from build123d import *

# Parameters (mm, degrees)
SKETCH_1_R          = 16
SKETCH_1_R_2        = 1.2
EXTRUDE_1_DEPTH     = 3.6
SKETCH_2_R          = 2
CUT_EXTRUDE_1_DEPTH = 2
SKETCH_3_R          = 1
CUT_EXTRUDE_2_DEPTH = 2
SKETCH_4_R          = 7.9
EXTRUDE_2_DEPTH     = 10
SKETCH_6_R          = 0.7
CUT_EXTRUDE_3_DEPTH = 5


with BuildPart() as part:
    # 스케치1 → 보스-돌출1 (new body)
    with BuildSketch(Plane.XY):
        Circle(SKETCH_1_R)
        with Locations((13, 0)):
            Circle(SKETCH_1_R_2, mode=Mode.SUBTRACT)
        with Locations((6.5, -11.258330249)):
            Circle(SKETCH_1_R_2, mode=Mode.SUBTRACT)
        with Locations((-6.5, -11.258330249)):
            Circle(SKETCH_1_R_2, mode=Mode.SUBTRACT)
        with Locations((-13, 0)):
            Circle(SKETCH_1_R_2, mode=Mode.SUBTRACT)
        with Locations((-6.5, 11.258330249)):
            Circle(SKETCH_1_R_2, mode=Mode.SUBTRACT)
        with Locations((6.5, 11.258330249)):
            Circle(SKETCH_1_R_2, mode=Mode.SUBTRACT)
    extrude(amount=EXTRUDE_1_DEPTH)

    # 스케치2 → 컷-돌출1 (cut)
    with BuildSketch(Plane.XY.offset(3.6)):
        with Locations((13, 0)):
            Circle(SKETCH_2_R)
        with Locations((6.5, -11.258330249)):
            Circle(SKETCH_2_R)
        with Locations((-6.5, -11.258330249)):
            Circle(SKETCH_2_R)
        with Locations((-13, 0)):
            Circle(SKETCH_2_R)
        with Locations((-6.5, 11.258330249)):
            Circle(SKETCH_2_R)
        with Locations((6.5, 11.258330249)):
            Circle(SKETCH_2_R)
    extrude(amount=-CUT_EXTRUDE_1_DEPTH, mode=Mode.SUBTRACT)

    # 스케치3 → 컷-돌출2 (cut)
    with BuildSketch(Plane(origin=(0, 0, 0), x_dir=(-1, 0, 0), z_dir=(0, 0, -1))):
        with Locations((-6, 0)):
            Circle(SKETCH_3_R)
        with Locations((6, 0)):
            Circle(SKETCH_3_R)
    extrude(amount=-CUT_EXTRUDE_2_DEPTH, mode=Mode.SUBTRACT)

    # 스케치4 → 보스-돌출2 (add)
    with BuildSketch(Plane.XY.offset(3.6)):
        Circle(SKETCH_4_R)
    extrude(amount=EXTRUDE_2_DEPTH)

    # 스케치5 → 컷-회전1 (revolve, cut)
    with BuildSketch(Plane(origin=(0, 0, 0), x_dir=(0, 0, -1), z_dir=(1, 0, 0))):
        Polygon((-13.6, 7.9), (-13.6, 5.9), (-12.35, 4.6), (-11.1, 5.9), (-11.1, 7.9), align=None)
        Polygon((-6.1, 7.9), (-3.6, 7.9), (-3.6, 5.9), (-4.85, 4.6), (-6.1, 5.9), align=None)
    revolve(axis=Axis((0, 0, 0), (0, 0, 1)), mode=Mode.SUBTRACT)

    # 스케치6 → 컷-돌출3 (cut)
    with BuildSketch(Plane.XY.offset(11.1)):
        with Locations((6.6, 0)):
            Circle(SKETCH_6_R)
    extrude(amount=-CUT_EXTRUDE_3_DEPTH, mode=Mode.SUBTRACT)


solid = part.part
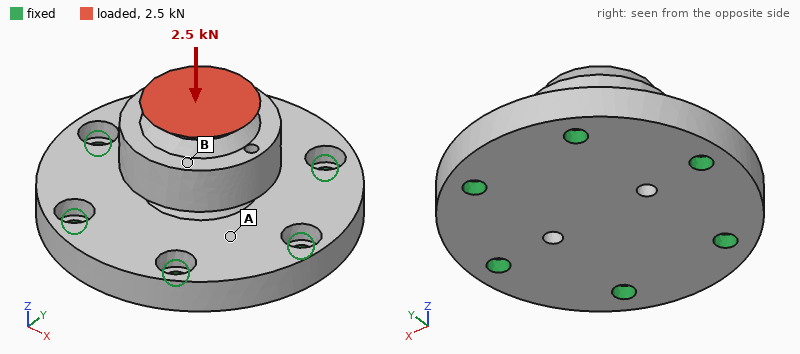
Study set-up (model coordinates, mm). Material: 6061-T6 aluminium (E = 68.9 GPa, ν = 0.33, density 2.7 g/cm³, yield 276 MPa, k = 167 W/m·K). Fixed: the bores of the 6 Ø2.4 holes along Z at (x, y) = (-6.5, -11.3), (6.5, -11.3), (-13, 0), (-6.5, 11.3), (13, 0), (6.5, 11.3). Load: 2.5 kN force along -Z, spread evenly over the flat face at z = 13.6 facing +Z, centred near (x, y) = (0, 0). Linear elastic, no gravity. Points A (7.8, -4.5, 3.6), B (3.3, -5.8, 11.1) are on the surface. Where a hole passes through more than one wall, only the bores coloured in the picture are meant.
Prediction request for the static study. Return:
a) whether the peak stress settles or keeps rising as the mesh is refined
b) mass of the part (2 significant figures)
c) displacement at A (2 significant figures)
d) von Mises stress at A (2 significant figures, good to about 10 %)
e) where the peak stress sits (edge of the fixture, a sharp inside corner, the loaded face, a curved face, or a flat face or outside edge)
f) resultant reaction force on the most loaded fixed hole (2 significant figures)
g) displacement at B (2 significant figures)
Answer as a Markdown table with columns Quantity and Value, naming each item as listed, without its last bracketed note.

| Quantity | Value |
|---|---|
| whether the peak stress settles or keeps rising as the mesh is refined | keeps rising |
| mass of the part | 11 g |
| displacement at A | 11 µm |
| von Mises stress at A | 41 MPa |
| where the peak stress sits | edge of the fixture |
| resultant reaction force on the most loaded fixed hole | 650 N |
| displacement at B | 24 µm |
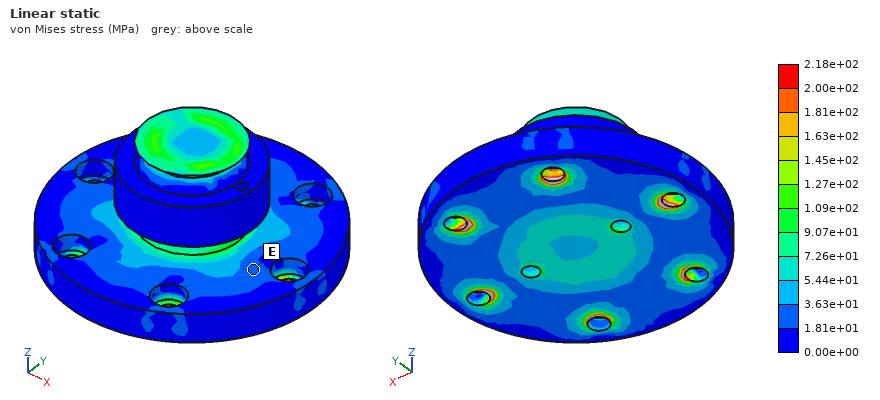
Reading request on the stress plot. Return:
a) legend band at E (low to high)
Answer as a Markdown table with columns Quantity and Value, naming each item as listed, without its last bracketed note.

| Quantity | Value |
|---|---|
| legend band at E | 1.81e+01 to 3.63e+01 MPa |
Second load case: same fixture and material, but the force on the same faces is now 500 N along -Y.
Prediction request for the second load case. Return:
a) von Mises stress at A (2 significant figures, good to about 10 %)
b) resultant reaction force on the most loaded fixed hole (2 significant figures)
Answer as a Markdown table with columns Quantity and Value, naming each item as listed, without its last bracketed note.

| Quantity | Value |
|---|---|
| von Mises stress at A | 13 MPa |
| resultant reaction force on the most loaded fixed hole | 220 N |
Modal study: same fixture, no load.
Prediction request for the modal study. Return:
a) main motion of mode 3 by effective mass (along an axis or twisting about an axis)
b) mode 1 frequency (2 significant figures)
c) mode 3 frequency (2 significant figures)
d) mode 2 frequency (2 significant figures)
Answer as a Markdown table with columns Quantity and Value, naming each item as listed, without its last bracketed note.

| Quantity | Value |
|---|---|
| main motion of mode 3 by effective mass | along Z |
| mode 1 frequency | 20 kHz |
| mode 3 frequency | 22 kHz |
| mode 2 frequency | 21 kHz |
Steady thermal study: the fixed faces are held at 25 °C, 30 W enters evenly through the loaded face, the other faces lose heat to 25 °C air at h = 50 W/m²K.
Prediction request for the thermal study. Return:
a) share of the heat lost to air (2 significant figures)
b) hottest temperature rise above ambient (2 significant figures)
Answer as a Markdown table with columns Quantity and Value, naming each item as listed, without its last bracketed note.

| Quantity | Value |
|---|---|
| share of the heat lost to air | 3.7 % |
| hottest temperature rise above ambient | 34 K |
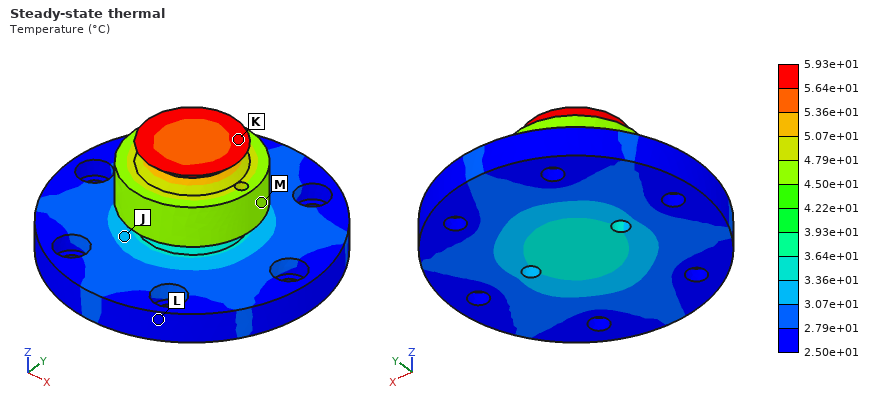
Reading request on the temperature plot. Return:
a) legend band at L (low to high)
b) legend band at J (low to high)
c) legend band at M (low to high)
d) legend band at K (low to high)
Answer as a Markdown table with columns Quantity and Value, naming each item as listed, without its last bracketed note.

| Quantity | Value |
|---|---|
| legend band at L | 2.50e+01 to 2.79e+01 °C |
| legend band at J | 3.07e+01 to 3.36e+01 °C |
| legend band at M | 4.50e+01 to 4.79e+01 °C |
| legend band at K | 5.64e+01 to 5.93e+01 °C |
